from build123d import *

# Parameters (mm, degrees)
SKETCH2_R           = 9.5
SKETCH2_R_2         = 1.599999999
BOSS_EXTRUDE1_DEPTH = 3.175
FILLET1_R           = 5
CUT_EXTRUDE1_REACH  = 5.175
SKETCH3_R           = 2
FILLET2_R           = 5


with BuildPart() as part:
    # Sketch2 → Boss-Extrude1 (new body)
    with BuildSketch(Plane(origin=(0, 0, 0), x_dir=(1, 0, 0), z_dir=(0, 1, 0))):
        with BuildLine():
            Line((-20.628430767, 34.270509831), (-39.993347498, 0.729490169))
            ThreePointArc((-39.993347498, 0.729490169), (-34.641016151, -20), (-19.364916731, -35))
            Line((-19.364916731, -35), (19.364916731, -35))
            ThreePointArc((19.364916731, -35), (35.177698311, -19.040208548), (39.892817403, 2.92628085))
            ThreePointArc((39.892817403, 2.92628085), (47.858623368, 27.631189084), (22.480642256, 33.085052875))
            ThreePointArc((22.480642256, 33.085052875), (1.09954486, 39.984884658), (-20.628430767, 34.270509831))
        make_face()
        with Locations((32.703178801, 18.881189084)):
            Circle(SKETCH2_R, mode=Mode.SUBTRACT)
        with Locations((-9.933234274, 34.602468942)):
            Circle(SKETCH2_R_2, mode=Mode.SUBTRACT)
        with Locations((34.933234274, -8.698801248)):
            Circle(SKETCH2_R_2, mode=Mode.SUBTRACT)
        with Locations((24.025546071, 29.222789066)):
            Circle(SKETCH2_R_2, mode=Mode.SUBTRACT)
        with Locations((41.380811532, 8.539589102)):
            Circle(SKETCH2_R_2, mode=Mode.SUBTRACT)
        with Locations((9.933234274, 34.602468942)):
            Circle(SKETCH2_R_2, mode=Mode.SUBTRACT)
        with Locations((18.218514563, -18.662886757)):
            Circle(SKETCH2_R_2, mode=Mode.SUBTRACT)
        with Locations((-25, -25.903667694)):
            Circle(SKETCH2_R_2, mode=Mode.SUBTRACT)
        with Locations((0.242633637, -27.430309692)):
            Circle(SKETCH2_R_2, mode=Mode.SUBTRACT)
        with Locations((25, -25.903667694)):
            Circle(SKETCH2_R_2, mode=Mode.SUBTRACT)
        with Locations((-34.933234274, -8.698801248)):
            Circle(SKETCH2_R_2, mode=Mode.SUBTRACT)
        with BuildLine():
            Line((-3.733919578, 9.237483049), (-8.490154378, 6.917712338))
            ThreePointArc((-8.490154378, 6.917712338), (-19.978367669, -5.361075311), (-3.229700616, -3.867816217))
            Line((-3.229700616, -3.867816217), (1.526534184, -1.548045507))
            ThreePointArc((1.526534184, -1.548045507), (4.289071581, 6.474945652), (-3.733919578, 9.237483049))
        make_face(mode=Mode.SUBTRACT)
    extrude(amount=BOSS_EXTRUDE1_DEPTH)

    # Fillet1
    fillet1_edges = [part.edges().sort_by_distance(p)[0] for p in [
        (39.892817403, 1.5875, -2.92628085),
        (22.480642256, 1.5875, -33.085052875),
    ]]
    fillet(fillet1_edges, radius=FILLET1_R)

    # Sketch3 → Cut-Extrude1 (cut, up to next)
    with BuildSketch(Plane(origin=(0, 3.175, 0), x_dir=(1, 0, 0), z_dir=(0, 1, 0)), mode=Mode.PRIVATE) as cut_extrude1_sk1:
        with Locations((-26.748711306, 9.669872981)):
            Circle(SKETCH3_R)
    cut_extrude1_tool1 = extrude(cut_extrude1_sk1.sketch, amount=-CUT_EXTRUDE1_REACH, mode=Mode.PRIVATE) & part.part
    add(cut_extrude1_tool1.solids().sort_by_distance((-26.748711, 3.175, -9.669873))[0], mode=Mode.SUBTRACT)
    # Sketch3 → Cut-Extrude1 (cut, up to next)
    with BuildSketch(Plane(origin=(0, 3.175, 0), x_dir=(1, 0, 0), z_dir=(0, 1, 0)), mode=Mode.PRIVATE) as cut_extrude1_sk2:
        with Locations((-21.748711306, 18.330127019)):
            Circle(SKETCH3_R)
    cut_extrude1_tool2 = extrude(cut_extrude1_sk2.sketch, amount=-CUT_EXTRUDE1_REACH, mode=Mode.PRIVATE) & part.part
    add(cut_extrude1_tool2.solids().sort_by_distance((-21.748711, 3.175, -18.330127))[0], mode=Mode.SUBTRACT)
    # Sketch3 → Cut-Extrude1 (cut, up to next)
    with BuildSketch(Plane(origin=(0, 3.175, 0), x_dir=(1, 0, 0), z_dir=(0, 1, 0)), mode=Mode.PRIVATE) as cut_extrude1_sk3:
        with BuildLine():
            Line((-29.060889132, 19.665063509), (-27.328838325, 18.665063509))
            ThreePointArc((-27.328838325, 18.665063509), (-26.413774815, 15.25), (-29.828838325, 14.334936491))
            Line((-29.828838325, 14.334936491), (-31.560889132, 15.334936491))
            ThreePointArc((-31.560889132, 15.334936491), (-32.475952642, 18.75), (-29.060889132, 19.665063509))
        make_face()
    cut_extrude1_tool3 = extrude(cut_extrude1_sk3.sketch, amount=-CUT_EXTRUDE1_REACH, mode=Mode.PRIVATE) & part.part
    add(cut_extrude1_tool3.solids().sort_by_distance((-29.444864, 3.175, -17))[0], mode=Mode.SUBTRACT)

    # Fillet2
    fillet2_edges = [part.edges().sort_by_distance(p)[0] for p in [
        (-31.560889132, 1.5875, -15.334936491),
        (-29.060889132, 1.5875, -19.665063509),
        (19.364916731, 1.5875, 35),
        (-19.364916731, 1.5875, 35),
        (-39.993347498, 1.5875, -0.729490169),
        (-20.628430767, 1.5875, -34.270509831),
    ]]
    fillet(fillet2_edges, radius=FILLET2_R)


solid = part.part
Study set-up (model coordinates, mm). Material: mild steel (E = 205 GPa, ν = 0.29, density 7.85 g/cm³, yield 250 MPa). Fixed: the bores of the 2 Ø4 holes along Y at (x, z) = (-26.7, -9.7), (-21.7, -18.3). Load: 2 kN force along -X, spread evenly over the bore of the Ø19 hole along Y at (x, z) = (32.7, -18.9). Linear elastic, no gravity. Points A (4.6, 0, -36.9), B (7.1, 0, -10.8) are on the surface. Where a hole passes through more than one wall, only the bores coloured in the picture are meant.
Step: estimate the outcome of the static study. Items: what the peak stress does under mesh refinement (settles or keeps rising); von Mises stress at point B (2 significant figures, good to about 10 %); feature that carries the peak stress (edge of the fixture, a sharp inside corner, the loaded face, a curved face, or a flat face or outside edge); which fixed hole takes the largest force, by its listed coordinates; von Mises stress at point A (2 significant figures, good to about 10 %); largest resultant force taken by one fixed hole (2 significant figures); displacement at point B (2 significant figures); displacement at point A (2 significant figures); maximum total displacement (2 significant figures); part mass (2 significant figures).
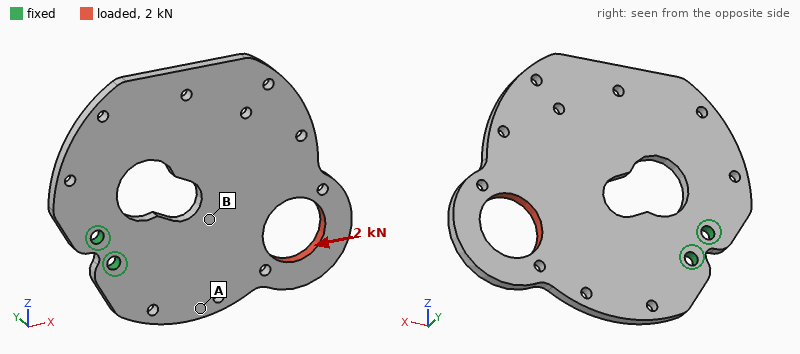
keeps rising
27 MPa
edge of the fixture
(-21.7, -18.3)
9.6 MPa
1.8 kN
6.5 µm
9.7 µm
19 µm
110 g
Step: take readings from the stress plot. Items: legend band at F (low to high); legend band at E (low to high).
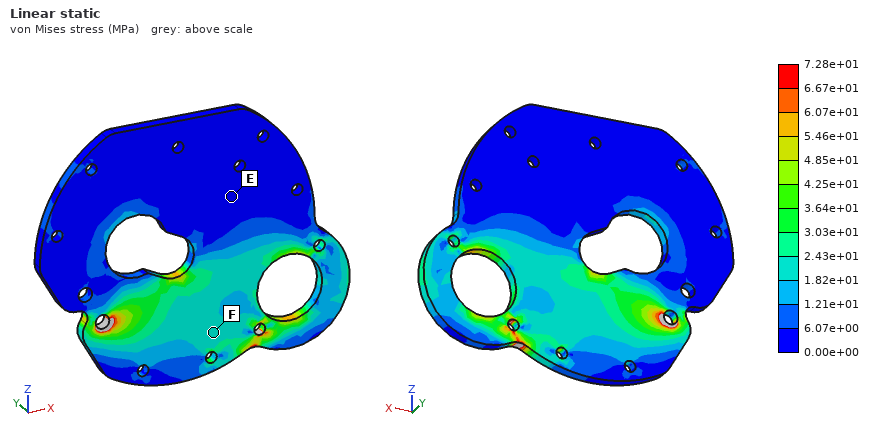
1.82e+01 to 2.43e+01 MPa
0.00e+00 to 6.07e+00 MPa
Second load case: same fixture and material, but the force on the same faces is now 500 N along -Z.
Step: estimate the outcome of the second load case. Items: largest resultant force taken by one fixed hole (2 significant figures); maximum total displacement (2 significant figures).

1.9 kN
51 µm
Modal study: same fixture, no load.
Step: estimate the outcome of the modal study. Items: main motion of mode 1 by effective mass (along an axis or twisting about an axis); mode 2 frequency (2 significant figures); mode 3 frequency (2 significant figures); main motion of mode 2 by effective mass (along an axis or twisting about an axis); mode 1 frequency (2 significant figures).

along Y
890 Hz
2100 Hz
twisting about X
480 Hz
